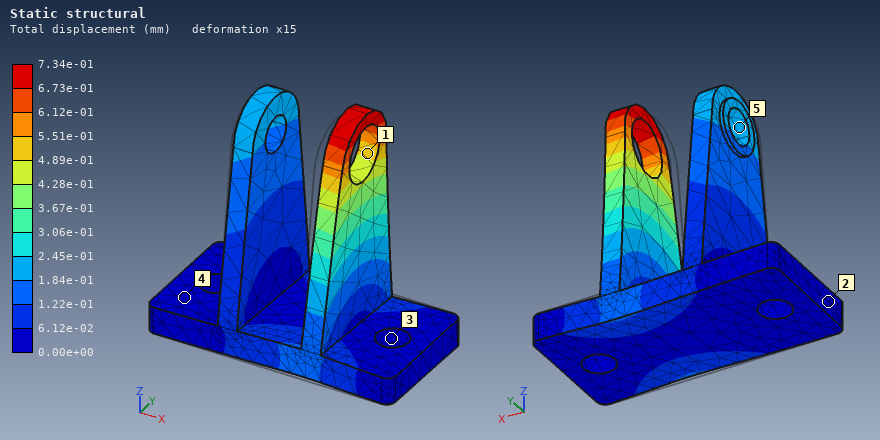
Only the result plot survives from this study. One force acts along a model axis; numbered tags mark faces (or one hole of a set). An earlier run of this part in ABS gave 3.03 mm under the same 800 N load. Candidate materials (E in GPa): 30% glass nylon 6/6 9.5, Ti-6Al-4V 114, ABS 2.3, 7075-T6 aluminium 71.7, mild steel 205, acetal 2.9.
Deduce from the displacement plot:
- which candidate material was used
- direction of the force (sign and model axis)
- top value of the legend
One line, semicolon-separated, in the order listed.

30% glass nylon 6/6; +Y; 7.34e-01 mm
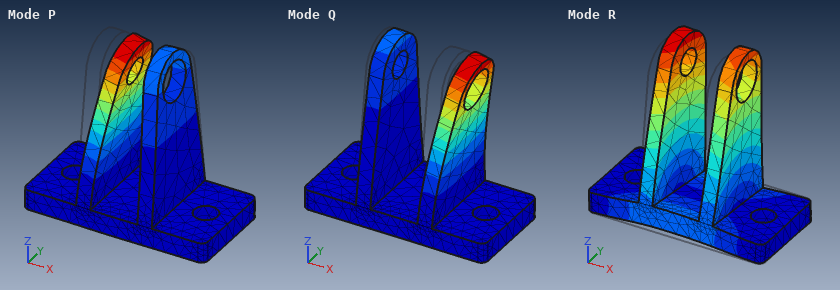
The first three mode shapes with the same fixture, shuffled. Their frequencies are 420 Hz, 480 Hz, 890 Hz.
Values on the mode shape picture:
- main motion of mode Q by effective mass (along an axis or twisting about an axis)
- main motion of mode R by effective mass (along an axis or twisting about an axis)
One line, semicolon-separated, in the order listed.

along X; along Y
